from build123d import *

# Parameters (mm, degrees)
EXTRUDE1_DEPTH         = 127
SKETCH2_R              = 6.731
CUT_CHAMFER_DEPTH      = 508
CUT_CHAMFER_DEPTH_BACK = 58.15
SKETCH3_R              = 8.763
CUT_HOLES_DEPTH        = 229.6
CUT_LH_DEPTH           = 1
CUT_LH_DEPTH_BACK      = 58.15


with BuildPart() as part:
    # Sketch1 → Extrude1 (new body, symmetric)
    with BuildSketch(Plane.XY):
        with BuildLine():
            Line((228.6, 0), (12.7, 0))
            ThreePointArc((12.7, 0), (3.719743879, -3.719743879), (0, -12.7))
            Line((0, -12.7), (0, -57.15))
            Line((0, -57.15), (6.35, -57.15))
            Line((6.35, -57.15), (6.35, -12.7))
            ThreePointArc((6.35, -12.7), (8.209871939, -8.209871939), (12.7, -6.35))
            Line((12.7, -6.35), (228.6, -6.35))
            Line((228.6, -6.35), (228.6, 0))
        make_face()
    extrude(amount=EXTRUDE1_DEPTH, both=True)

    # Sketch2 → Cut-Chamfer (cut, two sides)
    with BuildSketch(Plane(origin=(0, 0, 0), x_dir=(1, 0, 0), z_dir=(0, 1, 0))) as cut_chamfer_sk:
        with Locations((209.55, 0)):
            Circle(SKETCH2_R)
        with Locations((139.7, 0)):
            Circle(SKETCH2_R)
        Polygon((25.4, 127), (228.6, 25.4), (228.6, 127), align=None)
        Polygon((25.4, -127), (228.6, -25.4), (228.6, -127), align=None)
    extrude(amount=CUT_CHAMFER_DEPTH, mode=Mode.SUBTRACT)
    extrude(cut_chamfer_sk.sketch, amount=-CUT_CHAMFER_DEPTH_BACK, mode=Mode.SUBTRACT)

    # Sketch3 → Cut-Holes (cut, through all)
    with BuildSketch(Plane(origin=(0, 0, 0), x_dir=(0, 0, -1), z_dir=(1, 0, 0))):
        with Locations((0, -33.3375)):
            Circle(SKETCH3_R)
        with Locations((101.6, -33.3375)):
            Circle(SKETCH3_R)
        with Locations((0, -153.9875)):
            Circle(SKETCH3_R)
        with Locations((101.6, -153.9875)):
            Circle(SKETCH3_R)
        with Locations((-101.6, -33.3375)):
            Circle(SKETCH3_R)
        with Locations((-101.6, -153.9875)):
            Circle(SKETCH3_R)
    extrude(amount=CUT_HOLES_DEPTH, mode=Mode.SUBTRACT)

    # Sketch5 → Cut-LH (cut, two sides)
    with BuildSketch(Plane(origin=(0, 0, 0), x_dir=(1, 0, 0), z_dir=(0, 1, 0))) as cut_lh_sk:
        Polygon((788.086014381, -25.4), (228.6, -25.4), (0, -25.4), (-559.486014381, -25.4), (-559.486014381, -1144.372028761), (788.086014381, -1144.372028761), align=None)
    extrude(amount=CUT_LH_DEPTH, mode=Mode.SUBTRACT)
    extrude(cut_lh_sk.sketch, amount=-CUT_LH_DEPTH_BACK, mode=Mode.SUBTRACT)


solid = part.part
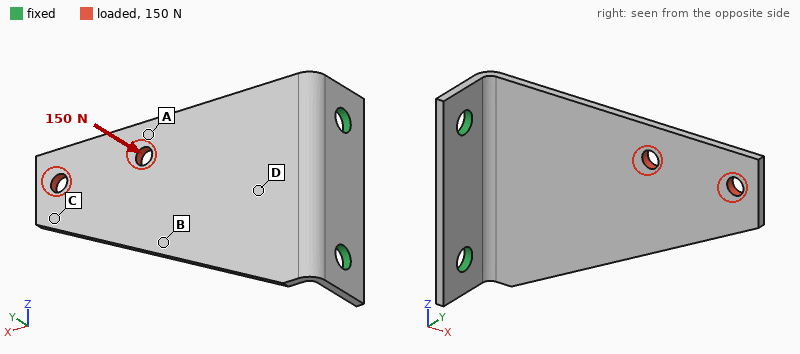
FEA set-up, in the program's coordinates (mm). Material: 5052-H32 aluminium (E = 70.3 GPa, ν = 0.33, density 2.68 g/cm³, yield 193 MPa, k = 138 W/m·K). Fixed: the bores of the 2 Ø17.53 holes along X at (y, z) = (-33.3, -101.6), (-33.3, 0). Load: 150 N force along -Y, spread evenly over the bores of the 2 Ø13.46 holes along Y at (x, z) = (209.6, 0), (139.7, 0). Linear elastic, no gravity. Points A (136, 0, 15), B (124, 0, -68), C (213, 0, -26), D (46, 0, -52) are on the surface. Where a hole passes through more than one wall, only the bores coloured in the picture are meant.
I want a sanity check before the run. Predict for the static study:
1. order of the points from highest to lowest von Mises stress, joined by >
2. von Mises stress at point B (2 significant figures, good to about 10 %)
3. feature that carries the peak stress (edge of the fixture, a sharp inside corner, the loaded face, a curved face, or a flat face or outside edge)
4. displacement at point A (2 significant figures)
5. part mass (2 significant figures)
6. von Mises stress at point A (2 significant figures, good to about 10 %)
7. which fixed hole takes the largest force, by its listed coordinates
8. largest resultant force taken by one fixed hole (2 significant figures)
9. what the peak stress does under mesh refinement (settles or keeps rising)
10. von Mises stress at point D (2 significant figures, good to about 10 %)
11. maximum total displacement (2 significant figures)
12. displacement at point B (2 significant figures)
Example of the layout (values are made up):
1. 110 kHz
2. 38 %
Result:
1. D > B > A > C
2. 15 MPa
3. edge of the fixture
4. 1.3 mm
5. 530 g
6. 11 MPa
7. (-33.3, 0)
8. 150 N
9. keeps rising
10. 19 MPa
11. 2.7 mm
12. 0.88 mm
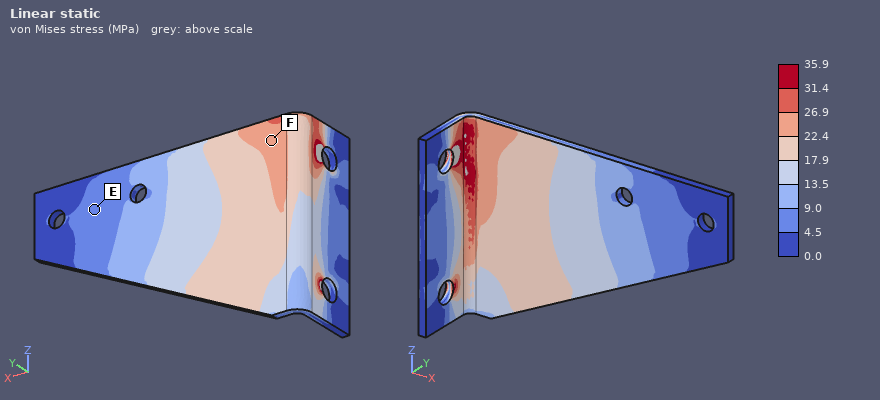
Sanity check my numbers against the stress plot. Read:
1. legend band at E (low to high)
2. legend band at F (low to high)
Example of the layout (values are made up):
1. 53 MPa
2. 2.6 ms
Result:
1. 4.5 to 9.0 MPa
2. 22.4 to 26.9 MPa
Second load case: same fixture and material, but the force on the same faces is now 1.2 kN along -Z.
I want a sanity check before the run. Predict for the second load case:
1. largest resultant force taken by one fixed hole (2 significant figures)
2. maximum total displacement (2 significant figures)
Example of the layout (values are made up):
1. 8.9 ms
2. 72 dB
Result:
1. 2.1 kN
2. 0.54 mm
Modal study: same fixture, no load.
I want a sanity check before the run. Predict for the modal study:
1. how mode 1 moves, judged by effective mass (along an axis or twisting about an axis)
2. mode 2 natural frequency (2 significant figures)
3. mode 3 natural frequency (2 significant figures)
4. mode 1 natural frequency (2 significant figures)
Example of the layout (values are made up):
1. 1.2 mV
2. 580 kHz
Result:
1. along Y
2. 570 Hz
3. 630 Hz
4. 120 Hz
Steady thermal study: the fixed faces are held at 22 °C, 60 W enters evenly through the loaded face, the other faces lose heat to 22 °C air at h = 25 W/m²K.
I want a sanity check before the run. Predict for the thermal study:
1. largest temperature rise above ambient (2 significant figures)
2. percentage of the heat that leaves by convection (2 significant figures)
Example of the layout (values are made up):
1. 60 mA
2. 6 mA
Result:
1. 75 K
2. 64 %
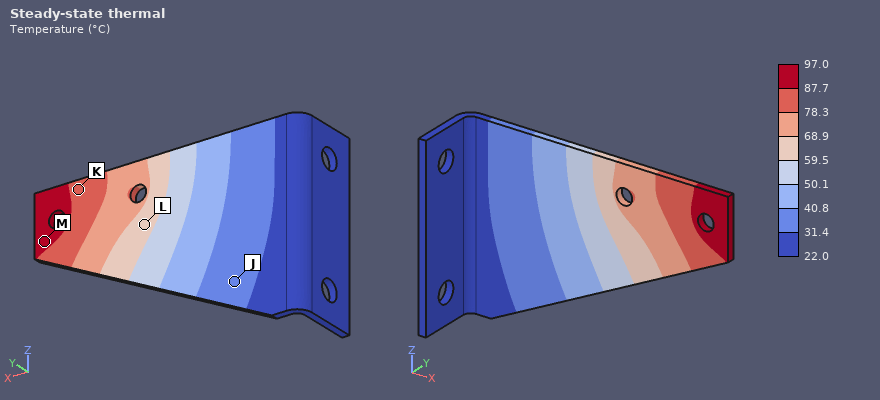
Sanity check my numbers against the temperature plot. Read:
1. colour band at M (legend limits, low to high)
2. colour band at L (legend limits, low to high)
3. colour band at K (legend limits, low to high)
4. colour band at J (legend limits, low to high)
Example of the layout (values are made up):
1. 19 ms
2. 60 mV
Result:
1. 87.7 to 97.0 °C
2. 59.5 to 68.9 °C
3. 78.3 to 87.7 °C
4. 31.4 to 40.8 °C
